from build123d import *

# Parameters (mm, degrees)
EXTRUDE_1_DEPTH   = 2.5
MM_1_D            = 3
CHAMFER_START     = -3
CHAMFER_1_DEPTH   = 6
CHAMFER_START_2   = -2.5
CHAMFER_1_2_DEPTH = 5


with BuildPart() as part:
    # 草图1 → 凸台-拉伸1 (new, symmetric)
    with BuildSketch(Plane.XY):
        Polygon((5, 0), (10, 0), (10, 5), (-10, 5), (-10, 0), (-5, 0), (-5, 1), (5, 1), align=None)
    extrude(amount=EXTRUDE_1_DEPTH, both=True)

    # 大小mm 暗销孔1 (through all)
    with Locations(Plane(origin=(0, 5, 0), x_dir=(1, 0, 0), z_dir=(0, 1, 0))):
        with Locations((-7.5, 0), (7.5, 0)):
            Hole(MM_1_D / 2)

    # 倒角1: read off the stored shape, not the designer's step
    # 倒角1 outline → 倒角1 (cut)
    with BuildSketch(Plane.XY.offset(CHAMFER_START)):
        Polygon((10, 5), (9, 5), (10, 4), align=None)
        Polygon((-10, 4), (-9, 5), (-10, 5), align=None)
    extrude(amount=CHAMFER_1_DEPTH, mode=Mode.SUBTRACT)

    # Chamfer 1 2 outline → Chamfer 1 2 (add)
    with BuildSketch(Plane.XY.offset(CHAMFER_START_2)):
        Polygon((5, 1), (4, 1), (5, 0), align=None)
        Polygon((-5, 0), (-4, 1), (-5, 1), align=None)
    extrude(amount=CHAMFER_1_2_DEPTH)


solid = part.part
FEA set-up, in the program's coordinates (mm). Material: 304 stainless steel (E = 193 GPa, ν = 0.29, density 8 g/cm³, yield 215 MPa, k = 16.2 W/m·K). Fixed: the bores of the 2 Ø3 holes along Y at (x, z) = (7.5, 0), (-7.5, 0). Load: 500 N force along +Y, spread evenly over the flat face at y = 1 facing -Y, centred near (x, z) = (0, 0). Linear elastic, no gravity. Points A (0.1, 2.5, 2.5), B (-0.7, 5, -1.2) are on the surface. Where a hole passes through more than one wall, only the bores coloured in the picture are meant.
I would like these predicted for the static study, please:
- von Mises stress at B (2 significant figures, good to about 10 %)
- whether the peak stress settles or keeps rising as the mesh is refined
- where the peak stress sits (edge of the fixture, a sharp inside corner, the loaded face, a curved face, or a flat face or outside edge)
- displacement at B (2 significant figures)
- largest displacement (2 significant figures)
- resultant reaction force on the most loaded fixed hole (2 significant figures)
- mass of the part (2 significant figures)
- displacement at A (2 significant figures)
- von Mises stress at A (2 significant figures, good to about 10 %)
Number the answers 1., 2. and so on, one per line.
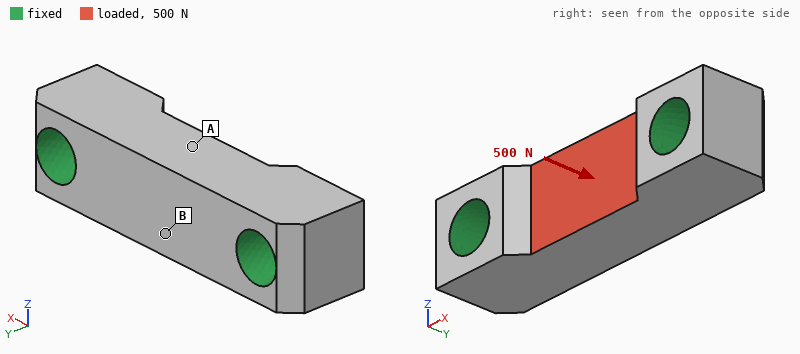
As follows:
1. 27 MPa
2. keeps rising
3. edge of the fixture
4. 1.2 µm
5. 1.4 µm
6. 250 N
7. 3.0 g
8. 1.4 µm
9. 7.7 MPa
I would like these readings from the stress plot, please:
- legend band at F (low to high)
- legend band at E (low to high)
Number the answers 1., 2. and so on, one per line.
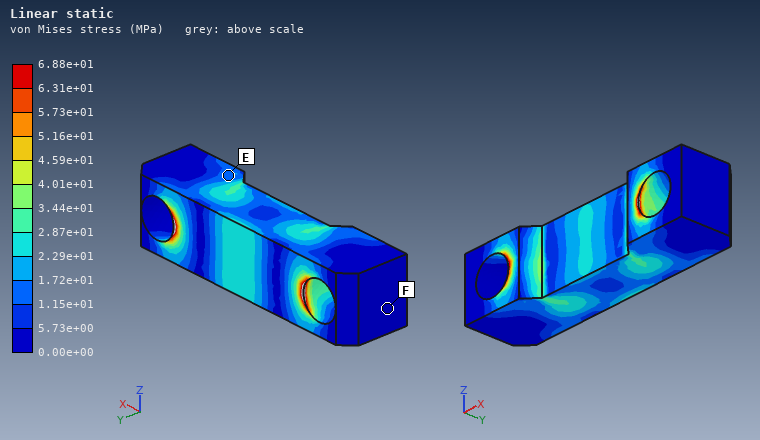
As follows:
1. 0.00e+00 to 5.73e+00 MPa
2. 1.15e+01 to 1.72e+01 MPa
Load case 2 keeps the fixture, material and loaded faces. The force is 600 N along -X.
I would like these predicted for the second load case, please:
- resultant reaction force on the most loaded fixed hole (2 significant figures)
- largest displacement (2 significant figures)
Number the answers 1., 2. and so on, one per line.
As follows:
1. 310 N
2. 0.66 µm
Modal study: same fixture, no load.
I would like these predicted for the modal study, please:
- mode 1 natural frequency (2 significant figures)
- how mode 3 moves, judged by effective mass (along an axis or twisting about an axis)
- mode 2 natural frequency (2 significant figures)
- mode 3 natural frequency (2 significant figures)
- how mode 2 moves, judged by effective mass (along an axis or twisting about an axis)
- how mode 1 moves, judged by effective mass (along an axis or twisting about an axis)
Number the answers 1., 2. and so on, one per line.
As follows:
1. 85 kHz
2. twisting about X
3. 92 kHz
4. 120 kHz
5. along Y
6. along Z
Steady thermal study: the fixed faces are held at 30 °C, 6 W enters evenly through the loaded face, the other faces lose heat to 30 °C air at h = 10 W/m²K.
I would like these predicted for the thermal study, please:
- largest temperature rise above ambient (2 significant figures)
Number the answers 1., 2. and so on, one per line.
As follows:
1. 49 K
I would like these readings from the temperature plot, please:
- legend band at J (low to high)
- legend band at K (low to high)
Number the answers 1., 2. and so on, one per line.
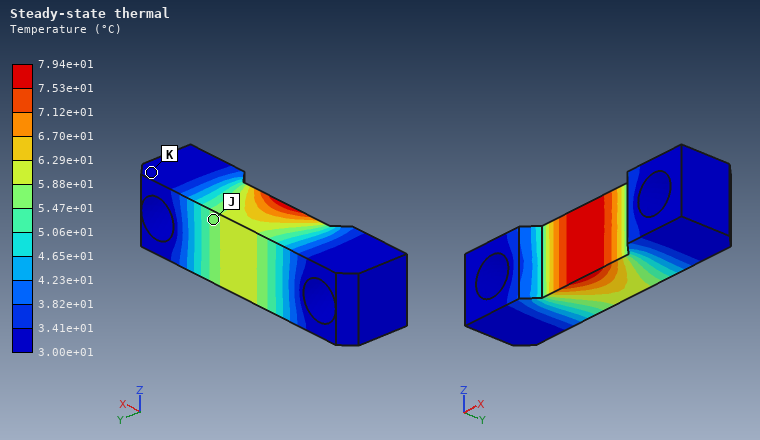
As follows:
1. 5.47e+01 to 5.88e+01 °C
2. 3.00e+01 to 3.41e+01 °C
